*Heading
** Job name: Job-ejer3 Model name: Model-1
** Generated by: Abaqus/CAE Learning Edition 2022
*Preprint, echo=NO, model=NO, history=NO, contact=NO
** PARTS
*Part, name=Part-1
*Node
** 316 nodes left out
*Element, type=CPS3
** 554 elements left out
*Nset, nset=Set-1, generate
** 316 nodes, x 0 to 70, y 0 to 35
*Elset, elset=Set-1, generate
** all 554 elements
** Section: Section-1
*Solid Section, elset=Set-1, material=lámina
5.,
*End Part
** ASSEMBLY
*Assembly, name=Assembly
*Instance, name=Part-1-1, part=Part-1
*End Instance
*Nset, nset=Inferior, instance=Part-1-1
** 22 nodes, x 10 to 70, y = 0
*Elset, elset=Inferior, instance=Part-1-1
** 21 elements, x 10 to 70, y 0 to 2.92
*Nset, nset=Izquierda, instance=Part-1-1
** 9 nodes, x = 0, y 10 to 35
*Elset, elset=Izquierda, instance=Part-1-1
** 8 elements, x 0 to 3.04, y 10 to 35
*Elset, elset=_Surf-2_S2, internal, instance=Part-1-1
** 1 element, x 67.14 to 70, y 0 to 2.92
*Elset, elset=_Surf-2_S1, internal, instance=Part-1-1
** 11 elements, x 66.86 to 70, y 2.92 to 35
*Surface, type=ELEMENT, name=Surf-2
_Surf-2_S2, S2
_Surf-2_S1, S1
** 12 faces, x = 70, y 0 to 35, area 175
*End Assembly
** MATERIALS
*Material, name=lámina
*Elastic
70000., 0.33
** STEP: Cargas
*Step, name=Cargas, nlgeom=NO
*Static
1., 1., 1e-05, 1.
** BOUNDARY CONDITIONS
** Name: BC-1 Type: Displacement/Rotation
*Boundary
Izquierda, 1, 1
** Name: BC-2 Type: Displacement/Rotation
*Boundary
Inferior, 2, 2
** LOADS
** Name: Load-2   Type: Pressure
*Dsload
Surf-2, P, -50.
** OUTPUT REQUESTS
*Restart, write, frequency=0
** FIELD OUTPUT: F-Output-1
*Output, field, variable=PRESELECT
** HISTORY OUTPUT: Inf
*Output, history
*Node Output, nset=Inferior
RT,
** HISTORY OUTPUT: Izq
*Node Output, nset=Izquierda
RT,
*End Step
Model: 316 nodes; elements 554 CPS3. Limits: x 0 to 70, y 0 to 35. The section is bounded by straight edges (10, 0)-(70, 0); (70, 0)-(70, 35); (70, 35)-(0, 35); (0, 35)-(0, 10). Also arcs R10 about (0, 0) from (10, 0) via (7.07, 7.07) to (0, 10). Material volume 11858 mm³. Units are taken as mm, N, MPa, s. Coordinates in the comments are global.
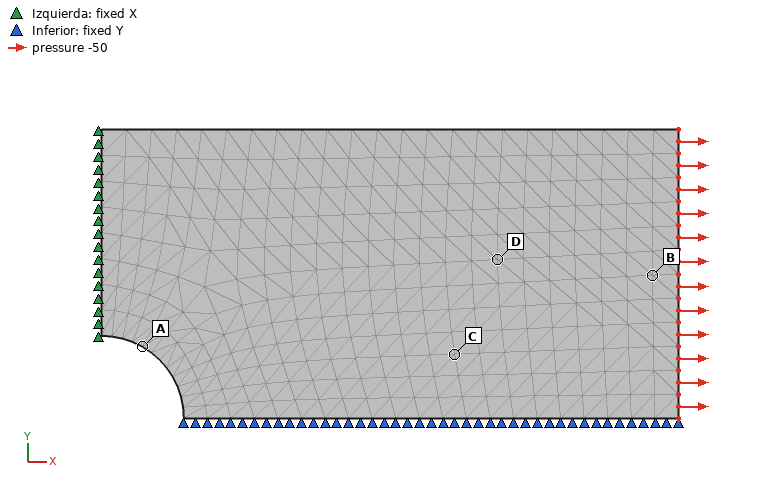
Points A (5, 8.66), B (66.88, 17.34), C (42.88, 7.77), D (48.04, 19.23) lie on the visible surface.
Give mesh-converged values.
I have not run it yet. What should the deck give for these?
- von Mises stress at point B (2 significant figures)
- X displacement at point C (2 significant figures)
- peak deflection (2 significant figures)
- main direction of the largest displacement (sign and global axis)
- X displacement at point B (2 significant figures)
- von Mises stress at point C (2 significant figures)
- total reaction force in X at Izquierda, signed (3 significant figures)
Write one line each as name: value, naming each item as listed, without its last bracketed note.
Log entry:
von Mises stress at point B: 49 MPa
X displacement at point C: 0.037 mm
peak deflection: 0.056 mm
main direction of the largest displacement: +X
X displacement at point B: 0.053 mm
von Mises stress at point C: 45 MPa
total reaction force in X at Izquierda, signed: -8750 N
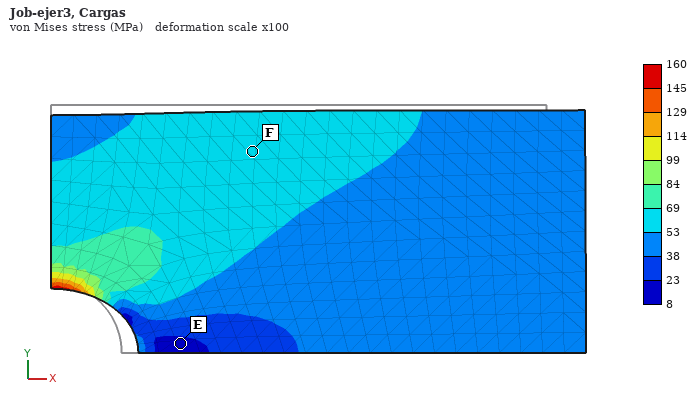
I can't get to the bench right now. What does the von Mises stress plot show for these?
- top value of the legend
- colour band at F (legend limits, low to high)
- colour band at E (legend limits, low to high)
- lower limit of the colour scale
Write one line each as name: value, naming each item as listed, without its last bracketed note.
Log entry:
top value of the legend: 160 MPa
colour band at F: 53 to 69 MPa
colour band at E: 8 to 23 MPa
lower limit of the colour scale: 8 MPa
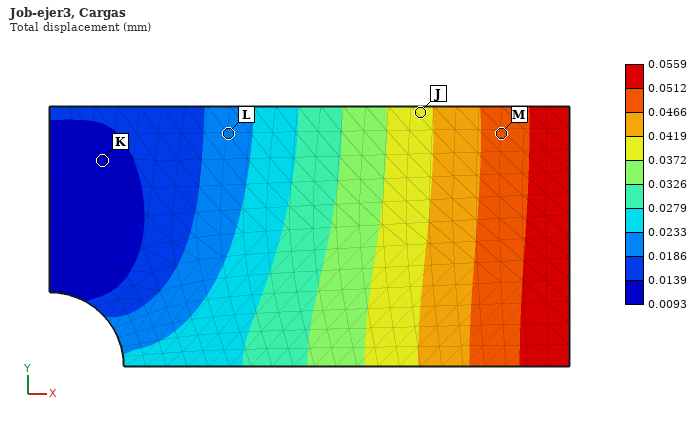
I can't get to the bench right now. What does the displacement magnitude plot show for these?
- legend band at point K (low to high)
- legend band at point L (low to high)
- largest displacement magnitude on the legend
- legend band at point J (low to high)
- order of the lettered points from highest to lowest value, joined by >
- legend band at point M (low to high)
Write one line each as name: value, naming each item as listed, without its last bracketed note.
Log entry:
legend band at point K: 0.0093 to 0.0139 mm
legend band at point L: 0.0186 to 0.0233 mm
largest displacement magnitude on the legend: 0.0559 mm
legend band at point J: 0.0372 to 0.0419 mm
order of the lettered points from highest to lowest value, joined by >: M > J > L > K
legend band at point M: 0.0466 to 0.0512 mm
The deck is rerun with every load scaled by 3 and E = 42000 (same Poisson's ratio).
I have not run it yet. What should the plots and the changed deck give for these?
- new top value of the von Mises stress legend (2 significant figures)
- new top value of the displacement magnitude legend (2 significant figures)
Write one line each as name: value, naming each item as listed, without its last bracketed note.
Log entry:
new top value of the von Mises stress legend: 480 MPa
new top value of the displacement magnitude legend: 0.28 mm
